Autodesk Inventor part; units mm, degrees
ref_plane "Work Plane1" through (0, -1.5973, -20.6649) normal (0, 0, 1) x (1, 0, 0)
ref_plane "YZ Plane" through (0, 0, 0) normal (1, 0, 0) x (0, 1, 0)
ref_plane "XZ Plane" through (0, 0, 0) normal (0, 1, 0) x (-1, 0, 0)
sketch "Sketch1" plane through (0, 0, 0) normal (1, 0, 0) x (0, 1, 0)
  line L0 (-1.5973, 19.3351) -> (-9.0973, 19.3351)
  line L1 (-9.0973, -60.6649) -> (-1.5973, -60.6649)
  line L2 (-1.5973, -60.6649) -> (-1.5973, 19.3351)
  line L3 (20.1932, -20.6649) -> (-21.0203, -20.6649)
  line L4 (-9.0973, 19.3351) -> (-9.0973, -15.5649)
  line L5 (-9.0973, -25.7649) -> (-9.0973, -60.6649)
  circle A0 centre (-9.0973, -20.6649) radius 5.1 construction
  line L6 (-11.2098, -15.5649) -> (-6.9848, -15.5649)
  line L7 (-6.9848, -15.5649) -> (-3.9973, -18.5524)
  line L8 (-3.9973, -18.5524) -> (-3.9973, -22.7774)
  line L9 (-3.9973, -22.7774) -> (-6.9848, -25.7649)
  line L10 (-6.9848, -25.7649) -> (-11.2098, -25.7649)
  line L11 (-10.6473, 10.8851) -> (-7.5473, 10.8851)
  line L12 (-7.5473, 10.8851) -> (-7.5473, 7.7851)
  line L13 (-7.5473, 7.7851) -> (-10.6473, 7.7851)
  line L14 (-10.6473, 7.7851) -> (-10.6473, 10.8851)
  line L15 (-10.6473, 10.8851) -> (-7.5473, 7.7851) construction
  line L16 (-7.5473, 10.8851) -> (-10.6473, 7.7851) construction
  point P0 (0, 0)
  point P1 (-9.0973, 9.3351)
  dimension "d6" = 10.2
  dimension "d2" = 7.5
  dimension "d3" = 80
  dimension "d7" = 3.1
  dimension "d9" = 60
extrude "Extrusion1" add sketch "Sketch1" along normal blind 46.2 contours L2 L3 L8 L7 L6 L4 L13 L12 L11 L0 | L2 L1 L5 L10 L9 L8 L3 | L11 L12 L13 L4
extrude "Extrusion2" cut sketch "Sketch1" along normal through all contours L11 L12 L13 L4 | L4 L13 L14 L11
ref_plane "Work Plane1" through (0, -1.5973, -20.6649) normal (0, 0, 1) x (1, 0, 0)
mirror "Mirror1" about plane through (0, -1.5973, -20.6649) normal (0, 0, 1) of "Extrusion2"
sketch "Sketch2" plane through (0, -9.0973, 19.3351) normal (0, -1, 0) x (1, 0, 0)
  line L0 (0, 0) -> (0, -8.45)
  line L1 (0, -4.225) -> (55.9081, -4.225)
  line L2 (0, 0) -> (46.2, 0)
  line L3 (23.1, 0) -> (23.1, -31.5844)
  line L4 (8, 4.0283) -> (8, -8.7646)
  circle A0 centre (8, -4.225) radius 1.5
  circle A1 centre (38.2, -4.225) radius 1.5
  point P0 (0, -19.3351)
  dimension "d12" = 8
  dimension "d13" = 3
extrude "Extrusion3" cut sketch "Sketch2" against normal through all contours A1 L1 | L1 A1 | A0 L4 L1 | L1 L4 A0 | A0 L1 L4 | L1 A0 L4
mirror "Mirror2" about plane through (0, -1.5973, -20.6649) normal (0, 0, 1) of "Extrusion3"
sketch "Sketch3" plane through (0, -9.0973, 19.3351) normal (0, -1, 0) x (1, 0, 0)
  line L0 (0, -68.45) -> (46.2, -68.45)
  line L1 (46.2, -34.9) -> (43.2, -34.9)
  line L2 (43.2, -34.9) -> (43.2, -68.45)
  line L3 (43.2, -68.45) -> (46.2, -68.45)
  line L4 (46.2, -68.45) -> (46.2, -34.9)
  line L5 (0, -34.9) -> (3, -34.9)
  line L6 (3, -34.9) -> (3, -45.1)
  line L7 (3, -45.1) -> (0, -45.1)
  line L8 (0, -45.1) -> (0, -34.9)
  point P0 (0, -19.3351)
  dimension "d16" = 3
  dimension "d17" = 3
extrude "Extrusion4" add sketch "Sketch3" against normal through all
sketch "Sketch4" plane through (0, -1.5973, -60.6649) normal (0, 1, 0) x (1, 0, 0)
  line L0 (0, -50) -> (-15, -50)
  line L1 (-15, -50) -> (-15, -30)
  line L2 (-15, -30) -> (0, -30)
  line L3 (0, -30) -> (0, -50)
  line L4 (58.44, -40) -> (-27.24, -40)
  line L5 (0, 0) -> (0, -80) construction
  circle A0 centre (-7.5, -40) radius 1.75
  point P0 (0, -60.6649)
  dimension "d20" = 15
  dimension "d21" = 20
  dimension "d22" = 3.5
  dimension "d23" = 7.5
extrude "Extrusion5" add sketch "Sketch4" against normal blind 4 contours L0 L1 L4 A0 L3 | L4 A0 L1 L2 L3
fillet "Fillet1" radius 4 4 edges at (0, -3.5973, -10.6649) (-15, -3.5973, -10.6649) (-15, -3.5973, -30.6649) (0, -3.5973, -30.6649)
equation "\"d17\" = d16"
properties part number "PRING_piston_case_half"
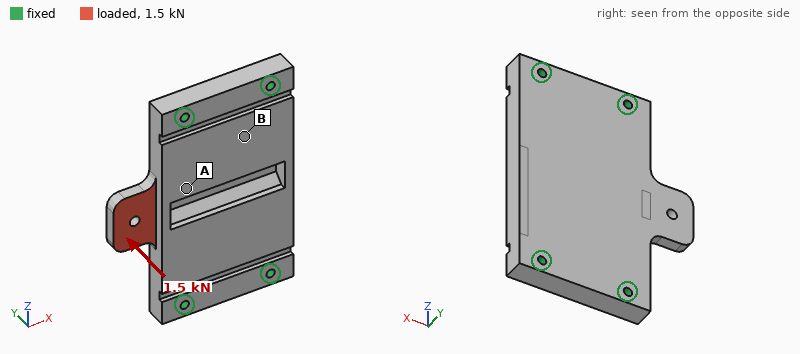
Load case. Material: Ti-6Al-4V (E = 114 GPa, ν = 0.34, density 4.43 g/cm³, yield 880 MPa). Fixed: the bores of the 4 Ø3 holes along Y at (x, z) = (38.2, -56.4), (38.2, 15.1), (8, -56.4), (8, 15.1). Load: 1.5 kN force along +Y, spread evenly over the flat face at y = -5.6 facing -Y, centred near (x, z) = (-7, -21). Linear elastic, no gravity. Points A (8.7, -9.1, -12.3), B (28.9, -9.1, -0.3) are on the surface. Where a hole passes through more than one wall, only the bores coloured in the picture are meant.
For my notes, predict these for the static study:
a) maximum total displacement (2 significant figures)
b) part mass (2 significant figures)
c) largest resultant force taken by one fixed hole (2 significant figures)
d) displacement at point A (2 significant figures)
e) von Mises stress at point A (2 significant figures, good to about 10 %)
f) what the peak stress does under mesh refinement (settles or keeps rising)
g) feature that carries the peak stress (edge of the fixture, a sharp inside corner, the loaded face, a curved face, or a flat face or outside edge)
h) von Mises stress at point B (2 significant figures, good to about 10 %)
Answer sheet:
0.23 mm
120 g
1.1 kN
0.054 mm
72 MPa
keeps rising
edge of the fixture
27 MPa
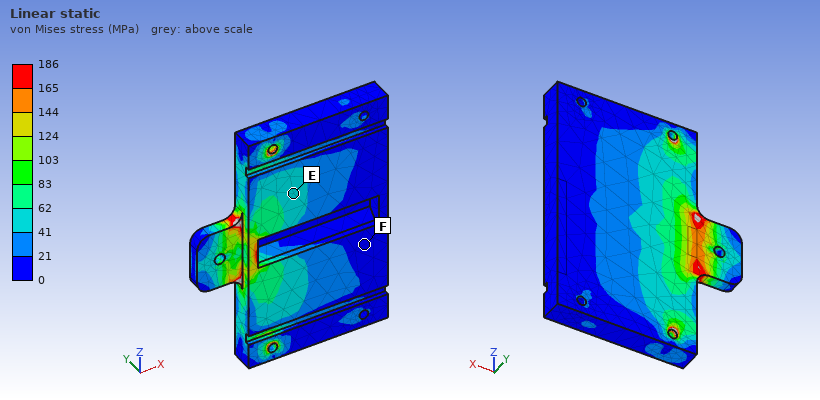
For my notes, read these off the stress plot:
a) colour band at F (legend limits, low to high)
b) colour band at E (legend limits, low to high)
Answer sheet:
0 to 21 MPa
41 to 62 MPa
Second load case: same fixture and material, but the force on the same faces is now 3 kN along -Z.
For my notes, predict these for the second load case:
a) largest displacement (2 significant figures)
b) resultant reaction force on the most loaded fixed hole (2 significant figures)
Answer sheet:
38 µm
1.2 kN
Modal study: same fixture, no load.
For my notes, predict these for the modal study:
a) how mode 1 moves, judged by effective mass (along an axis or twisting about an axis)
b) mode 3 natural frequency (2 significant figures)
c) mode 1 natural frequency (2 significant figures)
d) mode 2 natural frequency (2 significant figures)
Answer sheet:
along Y
12 kHz
4800 Hz
6800 Hz
